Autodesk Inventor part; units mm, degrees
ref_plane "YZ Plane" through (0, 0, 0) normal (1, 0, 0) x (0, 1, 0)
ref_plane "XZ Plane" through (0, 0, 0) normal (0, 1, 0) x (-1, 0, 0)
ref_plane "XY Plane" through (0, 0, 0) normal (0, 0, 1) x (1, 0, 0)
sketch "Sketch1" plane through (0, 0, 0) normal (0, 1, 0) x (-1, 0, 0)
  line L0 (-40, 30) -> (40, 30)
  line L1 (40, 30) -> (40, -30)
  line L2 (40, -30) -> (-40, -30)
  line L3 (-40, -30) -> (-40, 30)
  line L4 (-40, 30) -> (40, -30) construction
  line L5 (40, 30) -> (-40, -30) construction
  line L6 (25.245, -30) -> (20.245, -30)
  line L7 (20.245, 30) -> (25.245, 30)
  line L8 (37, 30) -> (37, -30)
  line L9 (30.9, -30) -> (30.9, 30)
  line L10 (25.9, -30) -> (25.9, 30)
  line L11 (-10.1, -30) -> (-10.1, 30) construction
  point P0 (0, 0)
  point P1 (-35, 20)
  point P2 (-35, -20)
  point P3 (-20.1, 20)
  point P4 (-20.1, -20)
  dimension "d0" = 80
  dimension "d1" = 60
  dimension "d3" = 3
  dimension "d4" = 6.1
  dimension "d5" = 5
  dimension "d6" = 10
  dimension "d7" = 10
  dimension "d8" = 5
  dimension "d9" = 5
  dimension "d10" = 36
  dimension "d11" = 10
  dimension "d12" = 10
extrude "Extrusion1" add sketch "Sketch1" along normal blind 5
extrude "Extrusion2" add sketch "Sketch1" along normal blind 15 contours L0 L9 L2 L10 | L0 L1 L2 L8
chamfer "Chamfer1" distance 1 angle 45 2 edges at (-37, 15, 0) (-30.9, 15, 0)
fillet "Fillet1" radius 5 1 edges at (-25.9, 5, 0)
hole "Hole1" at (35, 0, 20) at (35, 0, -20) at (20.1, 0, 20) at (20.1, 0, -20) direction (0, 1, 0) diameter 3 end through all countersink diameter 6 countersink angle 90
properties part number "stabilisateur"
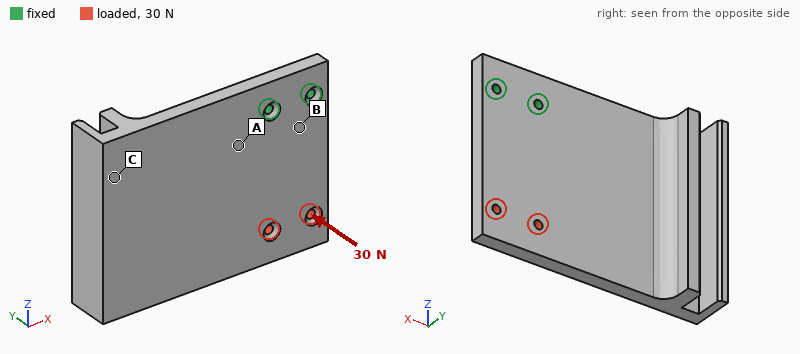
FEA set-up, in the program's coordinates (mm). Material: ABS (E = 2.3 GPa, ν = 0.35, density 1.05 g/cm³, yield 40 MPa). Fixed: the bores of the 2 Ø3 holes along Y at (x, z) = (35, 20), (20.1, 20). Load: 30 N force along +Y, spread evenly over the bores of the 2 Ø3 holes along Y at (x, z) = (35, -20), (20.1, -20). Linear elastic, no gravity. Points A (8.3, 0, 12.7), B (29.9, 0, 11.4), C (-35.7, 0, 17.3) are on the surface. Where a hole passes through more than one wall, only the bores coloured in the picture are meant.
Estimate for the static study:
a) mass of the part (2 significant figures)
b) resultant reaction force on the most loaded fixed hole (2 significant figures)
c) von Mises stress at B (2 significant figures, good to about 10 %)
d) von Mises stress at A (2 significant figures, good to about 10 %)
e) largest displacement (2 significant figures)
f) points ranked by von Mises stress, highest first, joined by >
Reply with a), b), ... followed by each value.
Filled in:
a) 30 g
b) 16 N
c) 5.6 MPa
d) 3.1 MPa
e) 1.2 mm
f) B > A > C
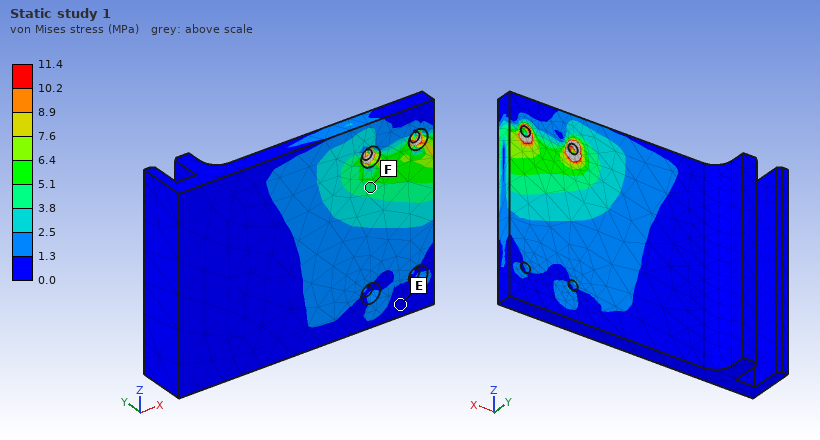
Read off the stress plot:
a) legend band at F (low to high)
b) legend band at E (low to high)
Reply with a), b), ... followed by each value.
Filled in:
a) 3.8 to 5.1 MPa
b) 0.0 to 1.3 MPa
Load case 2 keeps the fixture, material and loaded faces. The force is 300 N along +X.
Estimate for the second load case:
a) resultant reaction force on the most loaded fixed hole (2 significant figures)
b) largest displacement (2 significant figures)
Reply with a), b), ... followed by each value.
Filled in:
a) 740 N
b) 0.98 mm
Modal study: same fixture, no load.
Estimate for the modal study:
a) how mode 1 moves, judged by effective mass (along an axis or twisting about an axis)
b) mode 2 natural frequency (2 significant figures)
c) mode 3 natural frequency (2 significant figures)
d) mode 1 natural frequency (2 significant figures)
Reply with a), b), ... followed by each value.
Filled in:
a) along Y
b) 330 Hz
c) 630 Hz
d) 160 Hz
